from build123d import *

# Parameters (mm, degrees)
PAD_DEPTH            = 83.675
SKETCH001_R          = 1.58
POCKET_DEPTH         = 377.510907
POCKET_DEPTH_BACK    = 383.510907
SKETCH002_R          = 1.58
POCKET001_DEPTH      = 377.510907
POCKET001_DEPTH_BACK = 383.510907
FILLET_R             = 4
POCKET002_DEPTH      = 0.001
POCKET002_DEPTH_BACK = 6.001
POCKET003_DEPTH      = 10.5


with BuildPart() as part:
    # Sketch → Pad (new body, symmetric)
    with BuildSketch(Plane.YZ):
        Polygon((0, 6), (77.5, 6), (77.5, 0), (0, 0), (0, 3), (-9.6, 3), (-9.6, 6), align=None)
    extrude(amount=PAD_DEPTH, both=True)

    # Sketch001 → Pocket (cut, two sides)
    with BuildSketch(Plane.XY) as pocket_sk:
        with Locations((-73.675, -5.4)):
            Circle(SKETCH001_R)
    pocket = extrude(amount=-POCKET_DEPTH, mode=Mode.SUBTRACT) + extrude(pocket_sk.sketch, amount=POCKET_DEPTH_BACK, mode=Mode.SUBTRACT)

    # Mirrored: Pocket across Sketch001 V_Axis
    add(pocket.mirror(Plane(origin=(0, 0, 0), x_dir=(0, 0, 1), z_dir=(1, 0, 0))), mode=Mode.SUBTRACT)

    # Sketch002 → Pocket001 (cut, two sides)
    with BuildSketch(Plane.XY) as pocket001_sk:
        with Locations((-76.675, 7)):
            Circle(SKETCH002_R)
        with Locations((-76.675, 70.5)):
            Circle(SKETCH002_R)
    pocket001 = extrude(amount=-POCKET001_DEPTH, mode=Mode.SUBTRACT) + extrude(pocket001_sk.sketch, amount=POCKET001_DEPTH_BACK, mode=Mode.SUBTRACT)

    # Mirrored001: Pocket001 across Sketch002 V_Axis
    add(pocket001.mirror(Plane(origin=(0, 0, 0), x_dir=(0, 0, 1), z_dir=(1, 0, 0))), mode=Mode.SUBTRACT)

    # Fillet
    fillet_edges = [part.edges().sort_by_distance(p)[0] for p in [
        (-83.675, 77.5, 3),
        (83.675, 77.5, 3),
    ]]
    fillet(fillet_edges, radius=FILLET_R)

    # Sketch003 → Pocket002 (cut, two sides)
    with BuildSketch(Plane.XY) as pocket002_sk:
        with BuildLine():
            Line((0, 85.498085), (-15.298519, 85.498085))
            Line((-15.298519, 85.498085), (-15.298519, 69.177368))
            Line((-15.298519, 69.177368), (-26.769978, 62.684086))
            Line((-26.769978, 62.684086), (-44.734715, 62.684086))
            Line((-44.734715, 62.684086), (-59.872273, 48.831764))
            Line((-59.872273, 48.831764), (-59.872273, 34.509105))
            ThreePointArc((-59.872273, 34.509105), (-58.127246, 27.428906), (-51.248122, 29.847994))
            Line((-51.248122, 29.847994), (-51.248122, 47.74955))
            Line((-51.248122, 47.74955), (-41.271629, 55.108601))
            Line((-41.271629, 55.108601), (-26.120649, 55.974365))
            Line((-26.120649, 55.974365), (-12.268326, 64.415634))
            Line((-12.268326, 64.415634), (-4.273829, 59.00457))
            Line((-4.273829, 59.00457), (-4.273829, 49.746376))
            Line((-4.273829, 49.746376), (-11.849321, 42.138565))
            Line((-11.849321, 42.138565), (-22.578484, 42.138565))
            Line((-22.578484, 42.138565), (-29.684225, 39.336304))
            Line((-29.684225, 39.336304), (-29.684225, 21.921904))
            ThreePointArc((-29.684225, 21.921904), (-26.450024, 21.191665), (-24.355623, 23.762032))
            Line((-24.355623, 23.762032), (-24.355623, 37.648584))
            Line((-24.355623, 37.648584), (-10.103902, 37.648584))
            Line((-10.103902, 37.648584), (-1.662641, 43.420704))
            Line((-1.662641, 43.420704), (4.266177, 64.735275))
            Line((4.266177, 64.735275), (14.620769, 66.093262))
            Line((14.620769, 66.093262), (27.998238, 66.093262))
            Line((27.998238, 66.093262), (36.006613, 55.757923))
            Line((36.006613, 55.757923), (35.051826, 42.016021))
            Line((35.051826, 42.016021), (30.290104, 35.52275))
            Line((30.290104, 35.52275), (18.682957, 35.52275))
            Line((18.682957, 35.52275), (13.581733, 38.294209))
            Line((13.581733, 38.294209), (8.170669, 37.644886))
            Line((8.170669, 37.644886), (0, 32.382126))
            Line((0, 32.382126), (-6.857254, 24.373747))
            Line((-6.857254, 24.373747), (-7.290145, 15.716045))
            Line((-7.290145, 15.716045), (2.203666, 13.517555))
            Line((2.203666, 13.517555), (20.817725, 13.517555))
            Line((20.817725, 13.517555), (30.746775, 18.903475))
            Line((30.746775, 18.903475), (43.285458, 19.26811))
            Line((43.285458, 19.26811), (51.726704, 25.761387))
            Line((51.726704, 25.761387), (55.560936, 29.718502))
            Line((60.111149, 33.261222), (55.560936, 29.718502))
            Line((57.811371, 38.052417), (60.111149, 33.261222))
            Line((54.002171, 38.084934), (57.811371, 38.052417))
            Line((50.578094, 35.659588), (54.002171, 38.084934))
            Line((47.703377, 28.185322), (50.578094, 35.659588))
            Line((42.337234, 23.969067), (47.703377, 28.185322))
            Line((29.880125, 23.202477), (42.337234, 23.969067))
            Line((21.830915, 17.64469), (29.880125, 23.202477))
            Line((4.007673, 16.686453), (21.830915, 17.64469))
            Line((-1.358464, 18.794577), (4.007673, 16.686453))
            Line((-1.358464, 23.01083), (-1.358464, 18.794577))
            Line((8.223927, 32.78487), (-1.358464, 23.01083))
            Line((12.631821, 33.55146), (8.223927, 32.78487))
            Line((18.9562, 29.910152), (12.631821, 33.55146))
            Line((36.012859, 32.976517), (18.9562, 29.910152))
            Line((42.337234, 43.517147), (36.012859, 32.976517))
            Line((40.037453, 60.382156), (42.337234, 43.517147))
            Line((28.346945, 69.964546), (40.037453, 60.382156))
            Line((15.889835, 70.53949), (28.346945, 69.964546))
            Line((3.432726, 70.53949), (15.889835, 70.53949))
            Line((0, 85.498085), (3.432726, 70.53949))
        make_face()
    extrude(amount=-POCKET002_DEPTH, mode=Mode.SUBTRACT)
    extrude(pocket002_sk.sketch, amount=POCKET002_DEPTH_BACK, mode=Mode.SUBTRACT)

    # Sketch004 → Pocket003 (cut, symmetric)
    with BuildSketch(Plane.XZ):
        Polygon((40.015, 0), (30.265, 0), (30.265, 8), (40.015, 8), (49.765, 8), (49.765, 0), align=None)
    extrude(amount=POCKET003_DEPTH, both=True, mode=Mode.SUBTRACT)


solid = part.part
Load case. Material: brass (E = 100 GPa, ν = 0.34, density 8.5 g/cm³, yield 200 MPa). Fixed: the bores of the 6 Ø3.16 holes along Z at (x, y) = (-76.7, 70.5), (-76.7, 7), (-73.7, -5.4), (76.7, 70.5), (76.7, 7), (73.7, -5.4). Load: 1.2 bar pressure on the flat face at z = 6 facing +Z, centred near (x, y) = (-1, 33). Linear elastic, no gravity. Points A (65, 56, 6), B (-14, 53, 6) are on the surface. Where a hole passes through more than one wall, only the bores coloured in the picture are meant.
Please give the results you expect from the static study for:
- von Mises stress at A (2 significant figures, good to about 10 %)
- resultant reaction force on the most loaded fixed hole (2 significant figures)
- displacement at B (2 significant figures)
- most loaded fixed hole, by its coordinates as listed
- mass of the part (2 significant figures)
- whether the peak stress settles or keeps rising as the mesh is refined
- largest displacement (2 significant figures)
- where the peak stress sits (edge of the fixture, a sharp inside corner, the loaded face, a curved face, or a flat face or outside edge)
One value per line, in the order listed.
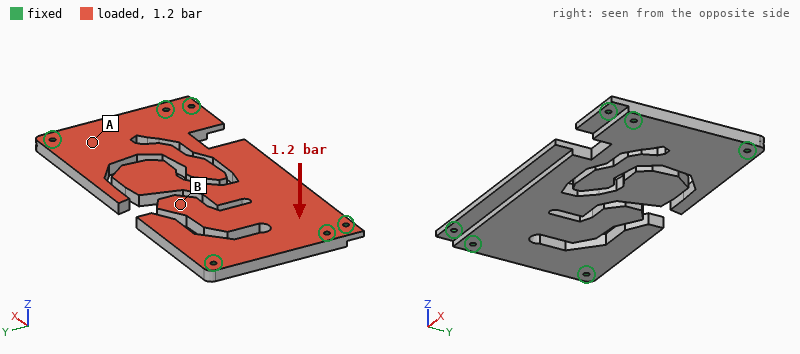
23 MPa
700 N
0.46 mm
(-76.7, 7)
580 g
keeps rising
1.00 mm
edge of the fixture
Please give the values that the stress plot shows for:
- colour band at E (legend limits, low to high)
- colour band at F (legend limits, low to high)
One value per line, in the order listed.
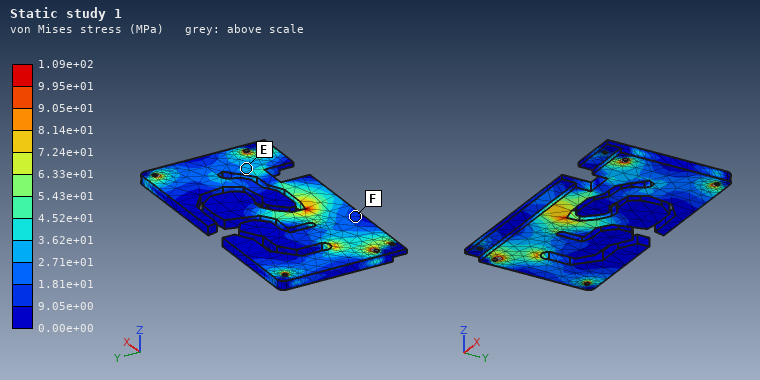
2.71e+01 to 3.62e+01 MPa
9.05e+00 to 1.81e+01 MPa
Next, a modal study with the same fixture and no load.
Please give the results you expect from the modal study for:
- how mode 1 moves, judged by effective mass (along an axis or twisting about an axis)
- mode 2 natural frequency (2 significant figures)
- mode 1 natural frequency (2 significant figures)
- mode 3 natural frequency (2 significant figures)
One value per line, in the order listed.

along Z
600 Hz
330 Hz
730 Hz
